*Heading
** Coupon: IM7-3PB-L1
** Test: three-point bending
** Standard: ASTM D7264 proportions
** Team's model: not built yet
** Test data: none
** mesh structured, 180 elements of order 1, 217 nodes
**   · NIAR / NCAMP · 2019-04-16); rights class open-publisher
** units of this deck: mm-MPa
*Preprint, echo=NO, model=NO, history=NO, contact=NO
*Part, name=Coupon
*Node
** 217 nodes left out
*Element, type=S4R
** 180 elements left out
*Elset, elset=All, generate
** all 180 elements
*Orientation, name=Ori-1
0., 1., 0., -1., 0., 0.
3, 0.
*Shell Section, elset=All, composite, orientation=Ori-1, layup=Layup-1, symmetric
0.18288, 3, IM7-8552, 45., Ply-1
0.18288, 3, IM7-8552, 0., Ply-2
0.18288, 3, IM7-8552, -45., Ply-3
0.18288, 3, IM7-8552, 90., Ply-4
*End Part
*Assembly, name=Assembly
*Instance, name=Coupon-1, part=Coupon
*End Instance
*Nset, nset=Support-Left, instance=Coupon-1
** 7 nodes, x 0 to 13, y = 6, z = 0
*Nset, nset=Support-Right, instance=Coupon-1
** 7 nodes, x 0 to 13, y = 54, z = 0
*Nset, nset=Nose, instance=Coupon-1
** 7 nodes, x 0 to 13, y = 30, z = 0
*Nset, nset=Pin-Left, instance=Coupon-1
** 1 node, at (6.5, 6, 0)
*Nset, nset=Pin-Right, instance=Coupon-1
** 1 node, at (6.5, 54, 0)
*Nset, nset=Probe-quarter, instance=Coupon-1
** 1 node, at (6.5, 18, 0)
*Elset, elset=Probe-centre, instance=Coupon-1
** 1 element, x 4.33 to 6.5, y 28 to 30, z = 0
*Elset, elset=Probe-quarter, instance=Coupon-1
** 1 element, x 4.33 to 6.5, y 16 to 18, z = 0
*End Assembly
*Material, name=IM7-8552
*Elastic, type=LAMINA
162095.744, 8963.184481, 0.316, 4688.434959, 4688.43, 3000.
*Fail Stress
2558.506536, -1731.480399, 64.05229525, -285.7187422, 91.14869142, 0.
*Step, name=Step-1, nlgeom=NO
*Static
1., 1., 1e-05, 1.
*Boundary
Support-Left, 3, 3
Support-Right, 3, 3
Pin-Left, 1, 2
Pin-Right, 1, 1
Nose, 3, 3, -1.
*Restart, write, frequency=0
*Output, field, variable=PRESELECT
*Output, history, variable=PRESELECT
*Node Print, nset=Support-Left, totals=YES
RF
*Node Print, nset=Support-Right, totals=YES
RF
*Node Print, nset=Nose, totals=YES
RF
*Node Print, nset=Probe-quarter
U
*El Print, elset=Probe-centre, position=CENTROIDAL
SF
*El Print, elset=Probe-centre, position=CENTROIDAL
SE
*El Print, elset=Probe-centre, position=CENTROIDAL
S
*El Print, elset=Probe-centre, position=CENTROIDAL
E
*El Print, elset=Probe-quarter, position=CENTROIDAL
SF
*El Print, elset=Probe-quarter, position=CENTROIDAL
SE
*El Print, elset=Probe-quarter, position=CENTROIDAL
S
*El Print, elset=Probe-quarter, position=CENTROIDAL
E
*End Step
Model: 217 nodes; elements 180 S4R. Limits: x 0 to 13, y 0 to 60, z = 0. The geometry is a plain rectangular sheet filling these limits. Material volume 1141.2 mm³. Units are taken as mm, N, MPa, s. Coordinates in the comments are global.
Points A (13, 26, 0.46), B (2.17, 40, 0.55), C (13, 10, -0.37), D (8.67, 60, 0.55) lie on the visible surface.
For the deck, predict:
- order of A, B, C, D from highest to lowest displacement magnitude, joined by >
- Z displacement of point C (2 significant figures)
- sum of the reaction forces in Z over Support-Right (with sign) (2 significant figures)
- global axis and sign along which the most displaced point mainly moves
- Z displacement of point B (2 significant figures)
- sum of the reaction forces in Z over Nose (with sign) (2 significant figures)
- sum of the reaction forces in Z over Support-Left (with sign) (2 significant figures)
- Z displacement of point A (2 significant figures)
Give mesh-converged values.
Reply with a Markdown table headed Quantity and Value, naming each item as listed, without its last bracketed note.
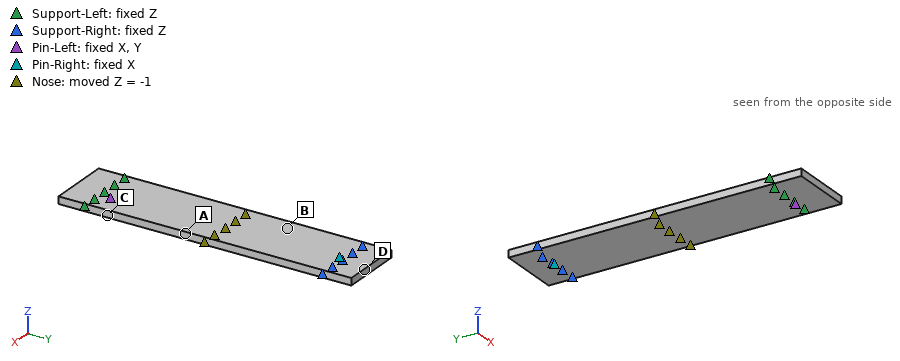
| Quantity | Value |
|---|---|
| order of A, B, C, D from highest to lowest displacement magnitude, joined by > | A > B > D > C |
| Z displacement of point C | -0.27 mm |
| sum of the reaction forces in Z over Support-Right (with sign) | 49 N |
| global axis and sign along which the most displaced point mainly moves | -Z |
| Z displacement of point B | -0.79 mm |
| sum of the reaction forces in Z over Nose (with sign) | -98 N |
| sum of the reaction forces in Z over Support-Left (with sign) | 49 N |
| Z displacement of point A | -0.99 mm |
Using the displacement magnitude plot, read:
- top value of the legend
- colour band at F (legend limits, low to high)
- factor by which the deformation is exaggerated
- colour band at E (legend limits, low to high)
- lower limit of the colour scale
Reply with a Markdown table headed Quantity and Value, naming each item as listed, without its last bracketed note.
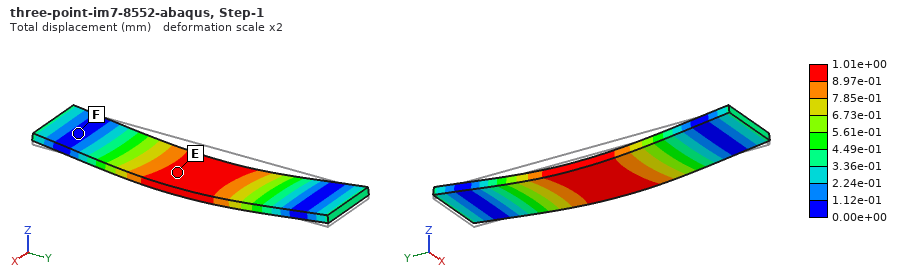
| Quantity | Value |
|---|---|
| top value of the legend | 1.01e+00 mm |
| colour band at F | 0.00e+00 to 1.12e-01 mm |
| factor by which the deformation is exaggerated | 2 |
| colour band at E | 8.97e-01 to 1.01e+00 mm |
| lower limit of the colour scale | 0.00e+00 mm |
